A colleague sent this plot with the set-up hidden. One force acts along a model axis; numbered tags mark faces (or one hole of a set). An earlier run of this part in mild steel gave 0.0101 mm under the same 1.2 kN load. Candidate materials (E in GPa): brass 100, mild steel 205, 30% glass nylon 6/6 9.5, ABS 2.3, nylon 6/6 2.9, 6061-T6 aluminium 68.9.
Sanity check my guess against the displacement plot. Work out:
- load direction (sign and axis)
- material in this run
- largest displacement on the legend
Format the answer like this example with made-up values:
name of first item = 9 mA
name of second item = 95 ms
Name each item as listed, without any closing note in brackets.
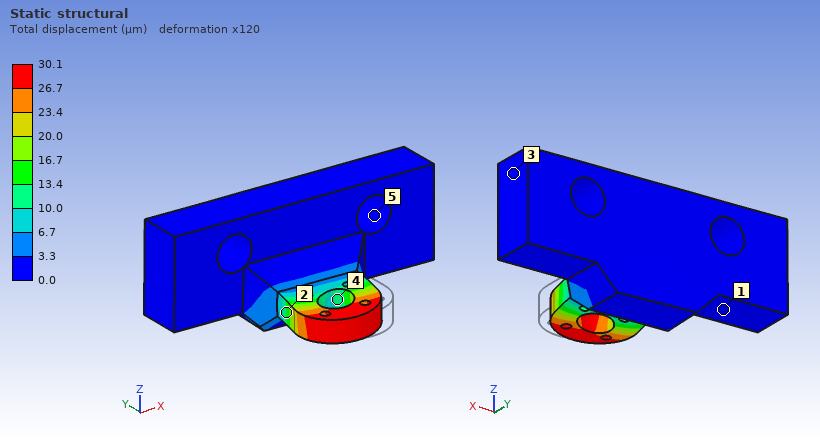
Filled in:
load direction = -X
material in this run = 6061-T6 aluminium
largest displacement on the legend = 30.1 µm
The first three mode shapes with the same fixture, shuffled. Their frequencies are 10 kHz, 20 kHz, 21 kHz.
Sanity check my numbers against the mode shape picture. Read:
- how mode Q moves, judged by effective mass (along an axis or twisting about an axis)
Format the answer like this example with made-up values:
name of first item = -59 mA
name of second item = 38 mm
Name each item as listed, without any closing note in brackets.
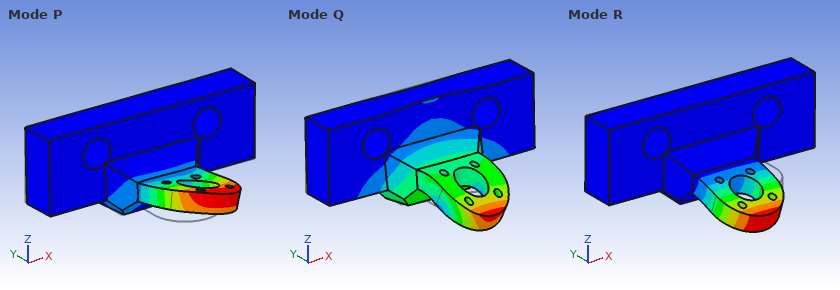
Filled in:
how mode Q moves, judged by effective mass = along Y
